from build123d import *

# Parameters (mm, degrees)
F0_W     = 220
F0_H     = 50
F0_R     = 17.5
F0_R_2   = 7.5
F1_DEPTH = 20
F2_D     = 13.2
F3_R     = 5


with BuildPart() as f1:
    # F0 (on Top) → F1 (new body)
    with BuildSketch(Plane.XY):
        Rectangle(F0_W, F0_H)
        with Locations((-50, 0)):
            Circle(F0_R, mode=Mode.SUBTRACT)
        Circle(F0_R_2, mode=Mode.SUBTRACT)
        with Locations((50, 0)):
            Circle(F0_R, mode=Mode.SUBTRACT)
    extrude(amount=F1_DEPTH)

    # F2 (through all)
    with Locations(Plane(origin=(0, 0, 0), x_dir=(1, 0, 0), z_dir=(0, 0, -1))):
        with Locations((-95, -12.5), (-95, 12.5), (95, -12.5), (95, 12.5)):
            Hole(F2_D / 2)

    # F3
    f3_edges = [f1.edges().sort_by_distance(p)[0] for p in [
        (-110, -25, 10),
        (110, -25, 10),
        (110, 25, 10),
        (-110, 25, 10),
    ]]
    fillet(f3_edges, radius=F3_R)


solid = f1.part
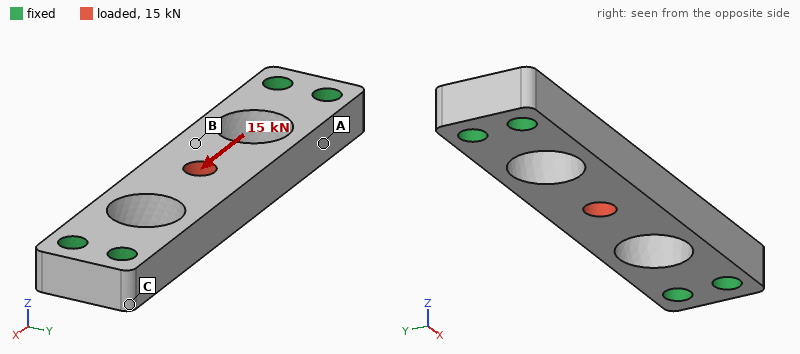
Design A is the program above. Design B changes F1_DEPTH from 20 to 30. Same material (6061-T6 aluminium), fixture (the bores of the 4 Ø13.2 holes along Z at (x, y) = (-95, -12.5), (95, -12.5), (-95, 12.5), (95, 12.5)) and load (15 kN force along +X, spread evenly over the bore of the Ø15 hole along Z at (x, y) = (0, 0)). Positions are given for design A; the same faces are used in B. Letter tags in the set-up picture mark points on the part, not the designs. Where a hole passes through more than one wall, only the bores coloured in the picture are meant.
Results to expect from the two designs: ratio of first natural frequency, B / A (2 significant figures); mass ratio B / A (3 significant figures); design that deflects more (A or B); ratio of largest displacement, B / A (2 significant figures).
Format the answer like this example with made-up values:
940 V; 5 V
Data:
1.2; 1.50; A; 0.66
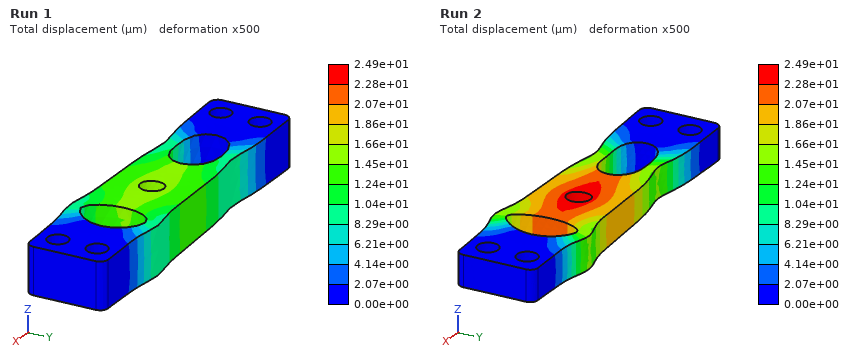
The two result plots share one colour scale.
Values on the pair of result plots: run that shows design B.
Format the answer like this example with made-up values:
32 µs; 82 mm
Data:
Run 1
